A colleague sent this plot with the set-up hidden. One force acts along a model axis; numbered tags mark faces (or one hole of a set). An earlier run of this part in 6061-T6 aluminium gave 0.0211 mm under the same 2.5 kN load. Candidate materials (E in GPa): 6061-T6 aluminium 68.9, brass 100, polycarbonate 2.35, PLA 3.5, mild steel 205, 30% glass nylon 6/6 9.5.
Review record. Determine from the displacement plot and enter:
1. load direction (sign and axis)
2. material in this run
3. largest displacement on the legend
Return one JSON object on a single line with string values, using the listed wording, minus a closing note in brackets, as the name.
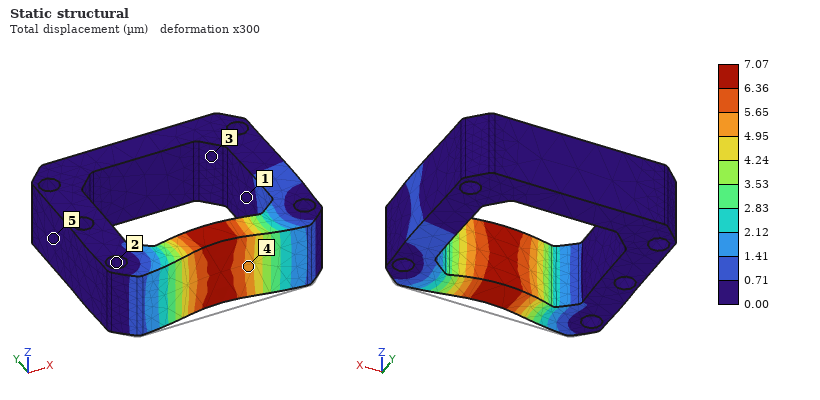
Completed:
{"load direction": "+Y", "material in this run": "mild steel", "largest displacement on the legend": "7.07 µm"}
